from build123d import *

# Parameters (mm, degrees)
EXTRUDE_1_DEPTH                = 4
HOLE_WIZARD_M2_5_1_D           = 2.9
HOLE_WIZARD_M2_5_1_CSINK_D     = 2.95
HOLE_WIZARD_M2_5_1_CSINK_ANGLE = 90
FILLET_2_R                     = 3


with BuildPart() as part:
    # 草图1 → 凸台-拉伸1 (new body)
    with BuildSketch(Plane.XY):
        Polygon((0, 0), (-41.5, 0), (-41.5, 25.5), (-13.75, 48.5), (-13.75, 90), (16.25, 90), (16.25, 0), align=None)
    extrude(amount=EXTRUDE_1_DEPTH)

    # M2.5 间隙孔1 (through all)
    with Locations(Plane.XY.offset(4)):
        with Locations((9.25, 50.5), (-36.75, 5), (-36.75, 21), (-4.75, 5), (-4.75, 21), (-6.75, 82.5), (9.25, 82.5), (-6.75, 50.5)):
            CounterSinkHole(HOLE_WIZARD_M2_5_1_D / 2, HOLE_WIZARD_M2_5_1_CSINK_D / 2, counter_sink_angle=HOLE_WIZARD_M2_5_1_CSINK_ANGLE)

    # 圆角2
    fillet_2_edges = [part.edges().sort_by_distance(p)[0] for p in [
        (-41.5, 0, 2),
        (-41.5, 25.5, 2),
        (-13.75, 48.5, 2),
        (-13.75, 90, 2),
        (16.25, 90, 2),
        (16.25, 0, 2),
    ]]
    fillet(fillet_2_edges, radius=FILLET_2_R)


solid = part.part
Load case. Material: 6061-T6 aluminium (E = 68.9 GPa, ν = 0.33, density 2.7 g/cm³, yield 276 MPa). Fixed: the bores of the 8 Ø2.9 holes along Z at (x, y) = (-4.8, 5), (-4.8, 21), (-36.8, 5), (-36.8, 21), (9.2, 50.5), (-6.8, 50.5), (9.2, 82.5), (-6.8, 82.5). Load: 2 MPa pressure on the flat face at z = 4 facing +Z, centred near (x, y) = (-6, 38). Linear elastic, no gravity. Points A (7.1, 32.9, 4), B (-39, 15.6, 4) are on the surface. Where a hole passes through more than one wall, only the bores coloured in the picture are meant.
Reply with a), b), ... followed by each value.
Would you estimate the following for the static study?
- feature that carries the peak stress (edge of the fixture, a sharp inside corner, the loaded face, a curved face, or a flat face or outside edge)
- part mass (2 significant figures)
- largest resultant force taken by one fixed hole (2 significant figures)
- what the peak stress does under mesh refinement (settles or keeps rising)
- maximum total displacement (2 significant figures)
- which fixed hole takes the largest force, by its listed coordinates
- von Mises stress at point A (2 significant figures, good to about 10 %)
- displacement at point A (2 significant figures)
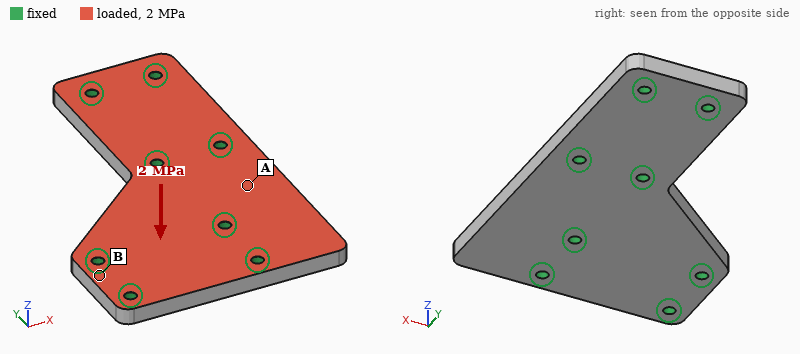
a) edge of the fixture
b) 40 g
c) 1.6 kN
d) keeps rising
e) 0.11 mm
f) (-4.8, 21)
g) 50 MPa
h) 0.039 mm
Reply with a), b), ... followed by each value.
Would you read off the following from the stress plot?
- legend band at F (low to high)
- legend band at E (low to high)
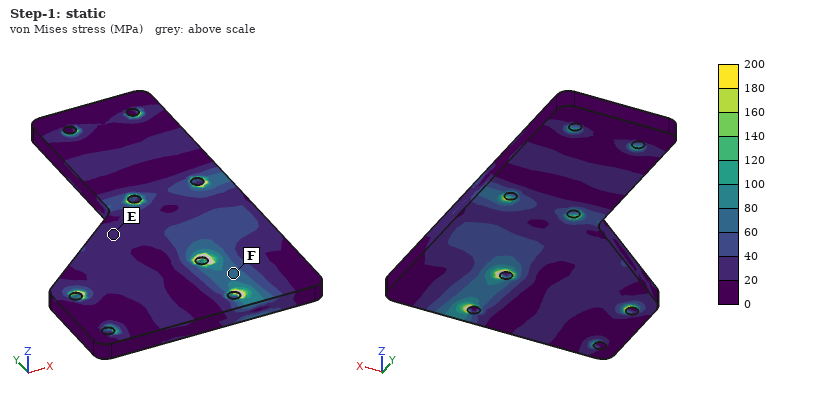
a) 60 to 80 MPa
b) 20 to 40 MPa
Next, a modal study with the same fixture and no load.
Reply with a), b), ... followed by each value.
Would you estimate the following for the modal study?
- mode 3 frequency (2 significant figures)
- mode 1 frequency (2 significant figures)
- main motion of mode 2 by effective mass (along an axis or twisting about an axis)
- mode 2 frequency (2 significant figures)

a) 14 kHz
b) 8100 Hz
c) along Z
d) 13 kHz
